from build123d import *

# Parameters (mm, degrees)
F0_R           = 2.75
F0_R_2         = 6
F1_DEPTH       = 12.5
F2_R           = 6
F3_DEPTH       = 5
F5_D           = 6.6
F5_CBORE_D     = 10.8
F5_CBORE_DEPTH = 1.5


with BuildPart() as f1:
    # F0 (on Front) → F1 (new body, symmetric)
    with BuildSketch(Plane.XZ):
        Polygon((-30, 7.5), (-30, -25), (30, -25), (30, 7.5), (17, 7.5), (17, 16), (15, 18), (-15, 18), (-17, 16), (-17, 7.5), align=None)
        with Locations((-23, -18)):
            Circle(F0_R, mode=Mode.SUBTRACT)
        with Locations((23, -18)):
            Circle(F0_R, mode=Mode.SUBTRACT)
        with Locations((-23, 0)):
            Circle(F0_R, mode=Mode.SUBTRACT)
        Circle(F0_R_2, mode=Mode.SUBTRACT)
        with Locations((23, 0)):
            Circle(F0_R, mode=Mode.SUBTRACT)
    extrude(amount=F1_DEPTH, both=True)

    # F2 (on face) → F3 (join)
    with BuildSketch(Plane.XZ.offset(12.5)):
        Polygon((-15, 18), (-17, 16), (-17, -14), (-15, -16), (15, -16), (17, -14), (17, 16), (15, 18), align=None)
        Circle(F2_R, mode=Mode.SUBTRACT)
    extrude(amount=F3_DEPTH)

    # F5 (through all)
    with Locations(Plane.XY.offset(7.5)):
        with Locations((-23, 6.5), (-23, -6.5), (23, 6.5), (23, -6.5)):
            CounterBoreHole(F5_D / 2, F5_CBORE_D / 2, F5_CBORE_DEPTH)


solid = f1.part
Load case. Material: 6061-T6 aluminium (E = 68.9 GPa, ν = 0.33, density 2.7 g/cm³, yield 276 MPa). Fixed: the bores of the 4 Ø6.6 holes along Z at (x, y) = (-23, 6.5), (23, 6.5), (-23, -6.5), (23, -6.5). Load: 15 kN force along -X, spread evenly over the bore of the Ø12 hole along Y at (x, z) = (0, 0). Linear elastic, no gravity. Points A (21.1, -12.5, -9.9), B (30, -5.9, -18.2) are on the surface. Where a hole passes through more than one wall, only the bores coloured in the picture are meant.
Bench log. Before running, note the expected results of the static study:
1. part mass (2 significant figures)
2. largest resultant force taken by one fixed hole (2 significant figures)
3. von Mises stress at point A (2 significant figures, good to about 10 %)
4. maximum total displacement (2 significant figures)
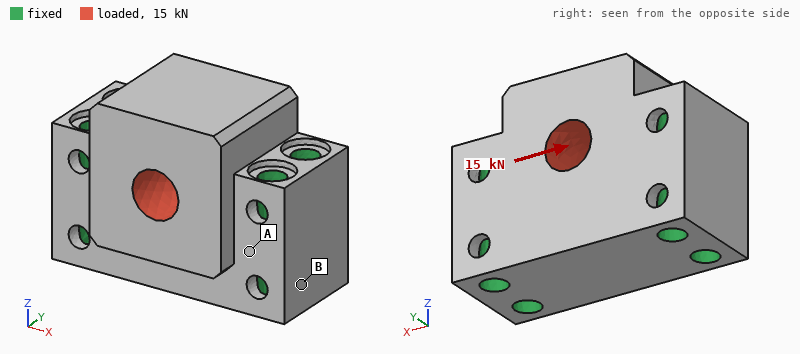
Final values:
150 g
4.2 kN
7.4 MPa
5.5 µm
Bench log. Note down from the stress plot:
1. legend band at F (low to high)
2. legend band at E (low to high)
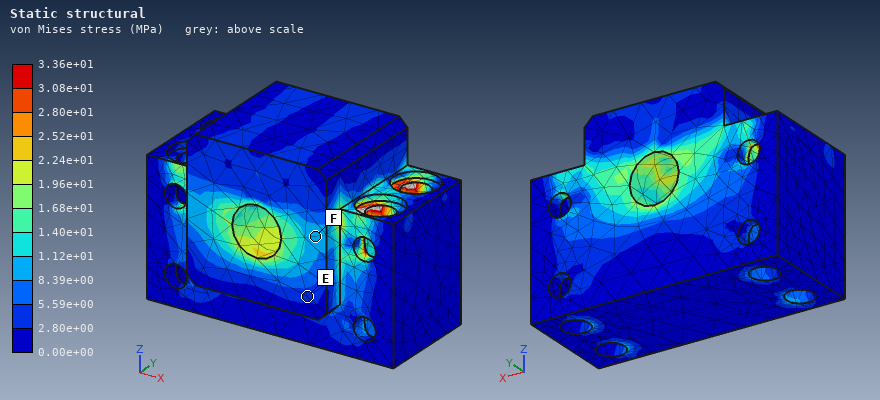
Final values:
8.39e+00 to 1.12e+01 MPa
2.80e+00 to 5.59e+00 MPa
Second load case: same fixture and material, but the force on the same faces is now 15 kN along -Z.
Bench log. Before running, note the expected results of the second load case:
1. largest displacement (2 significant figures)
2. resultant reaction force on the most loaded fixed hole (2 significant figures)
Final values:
9.8 µm
4.5 kN
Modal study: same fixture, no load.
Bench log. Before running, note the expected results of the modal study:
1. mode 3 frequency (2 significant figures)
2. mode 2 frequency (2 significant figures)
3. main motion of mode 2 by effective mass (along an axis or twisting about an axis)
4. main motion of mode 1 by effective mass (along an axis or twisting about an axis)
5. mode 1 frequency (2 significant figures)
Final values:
31 kHz
29 kHz
along Z
along Y
19 kHz
